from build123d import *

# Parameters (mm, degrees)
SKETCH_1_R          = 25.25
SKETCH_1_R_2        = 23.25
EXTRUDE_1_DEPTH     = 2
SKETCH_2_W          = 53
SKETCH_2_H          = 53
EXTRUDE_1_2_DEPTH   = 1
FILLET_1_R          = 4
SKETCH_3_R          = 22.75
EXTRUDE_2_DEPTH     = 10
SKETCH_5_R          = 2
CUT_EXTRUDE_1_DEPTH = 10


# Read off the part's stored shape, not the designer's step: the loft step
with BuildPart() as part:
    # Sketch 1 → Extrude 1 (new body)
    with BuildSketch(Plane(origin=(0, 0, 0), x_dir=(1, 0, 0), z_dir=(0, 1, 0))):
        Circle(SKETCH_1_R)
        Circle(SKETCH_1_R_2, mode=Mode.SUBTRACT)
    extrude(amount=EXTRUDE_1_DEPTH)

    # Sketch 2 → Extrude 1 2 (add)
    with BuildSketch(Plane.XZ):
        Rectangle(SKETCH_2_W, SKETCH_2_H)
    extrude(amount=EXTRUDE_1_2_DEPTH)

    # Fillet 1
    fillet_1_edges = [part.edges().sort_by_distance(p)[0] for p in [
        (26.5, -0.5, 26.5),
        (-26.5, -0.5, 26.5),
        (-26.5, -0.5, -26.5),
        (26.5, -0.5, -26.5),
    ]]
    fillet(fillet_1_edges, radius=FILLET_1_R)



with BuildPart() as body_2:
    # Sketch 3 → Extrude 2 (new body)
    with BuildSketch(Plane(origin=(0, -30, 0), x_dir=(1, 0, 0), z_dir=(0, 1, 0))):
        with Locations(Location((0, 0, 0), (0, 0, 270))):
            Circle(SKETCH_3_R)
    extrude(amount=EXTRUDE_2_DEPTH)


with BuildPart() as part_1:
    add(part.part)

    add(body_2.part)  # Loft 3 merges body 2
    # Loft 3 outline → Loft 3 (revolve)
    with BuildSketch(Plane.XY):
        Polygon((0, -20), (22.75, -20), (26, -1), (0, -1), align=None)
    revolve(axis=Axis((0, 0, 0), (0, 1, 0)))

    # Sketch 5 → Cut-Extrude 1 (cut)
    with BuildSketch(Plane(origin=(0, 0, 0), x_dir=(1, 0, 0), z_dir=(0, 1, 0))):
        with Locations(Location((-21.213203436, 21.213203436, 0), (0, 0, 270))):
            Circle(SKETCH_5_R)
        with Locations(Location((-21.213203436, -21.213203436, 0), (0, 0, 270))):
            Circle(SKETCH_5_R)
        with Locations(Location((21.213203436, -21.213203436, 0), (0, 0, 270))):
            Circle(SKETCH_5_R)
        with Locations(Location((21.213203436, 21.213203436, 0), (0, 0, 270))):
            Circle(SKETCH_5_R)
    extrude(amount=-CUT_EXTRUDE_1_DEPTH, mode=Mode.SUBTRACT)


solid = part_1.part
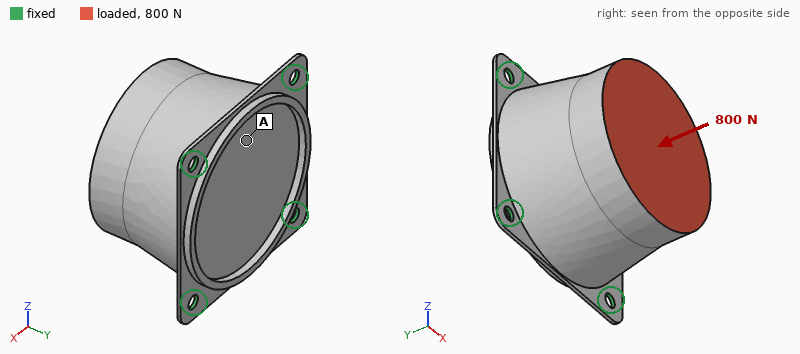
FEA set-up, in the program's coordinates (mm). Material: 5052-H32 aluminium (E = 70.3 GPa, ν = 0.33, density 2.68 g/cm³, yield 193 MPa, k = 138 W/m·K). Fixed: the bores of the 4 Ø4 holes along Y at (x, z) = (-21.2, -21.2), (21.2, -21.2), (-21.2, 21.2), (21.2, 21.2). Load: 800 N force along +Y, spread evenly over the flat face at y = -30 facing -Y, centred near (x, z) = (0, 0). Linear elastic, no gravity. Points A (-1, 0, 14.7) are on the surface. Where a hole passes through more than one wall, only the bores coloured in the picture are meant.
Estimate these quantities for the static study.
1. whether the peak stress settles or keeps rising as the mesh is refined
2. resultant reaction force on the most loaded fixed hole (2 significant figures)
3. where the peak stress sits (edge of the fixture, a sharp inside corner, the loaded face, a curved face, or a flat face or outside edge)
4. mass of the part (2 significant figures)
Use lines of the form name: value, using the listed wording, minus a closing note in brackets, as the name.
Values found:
whether the peak stress settles or keeps rising as the mesh is refined: keeps rising
resultant reaction force on the most loaded fixed hole: 230 N
where the peak stress sits: edge of the fixture
mass of the part: 150 g
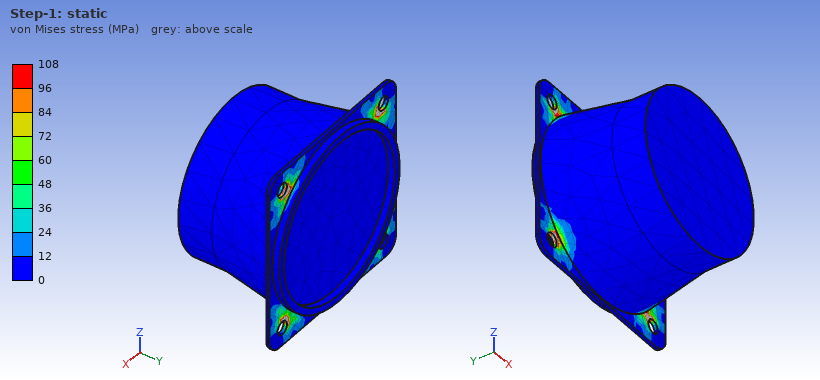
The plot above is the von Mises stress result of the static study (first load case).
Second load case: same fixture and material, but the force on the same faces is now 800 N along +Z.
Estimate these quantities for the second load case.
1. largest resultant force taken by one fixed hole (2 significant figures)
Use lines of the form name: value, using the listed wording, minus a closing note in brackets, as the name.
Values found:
largest resultant force taken by one fixed hole: 390 N
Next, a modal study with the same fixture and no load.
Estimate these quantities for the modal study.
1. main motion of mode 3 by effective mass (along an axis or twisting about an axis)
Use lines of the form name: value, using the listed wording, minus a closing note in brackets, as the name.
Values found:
main motion of mode 3 by effective mass: along Y
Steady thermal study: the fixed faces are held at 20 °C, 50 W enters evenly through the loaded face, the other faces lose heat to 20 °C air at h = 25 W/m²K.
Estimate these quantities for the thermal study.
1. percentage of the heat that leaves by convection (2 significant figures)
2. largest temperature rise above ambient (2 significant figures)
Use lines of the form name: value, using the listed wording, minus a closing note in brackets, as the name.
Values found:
percentage of the heat that leaves by convection: 12 %
largest temperature rise above ambient: 35 K
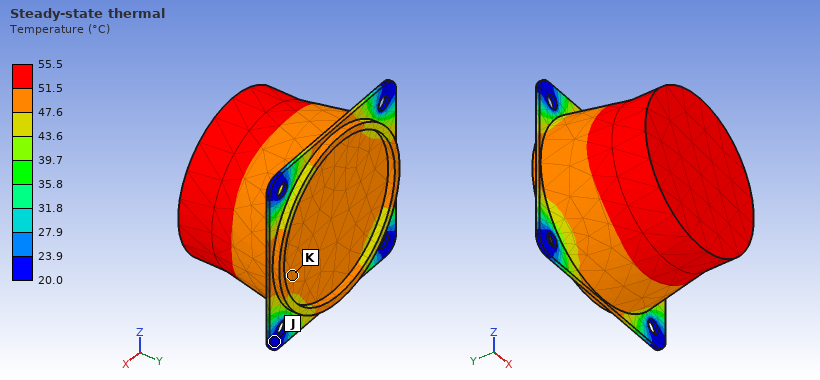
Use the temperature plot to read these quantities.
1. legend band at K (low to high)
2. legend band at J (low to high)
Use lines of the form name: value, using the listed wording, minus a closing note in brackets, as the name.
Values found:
legend band at K: 47.6 to 51.5 °C
legend band at J: 20.0 to 23.9 °C
